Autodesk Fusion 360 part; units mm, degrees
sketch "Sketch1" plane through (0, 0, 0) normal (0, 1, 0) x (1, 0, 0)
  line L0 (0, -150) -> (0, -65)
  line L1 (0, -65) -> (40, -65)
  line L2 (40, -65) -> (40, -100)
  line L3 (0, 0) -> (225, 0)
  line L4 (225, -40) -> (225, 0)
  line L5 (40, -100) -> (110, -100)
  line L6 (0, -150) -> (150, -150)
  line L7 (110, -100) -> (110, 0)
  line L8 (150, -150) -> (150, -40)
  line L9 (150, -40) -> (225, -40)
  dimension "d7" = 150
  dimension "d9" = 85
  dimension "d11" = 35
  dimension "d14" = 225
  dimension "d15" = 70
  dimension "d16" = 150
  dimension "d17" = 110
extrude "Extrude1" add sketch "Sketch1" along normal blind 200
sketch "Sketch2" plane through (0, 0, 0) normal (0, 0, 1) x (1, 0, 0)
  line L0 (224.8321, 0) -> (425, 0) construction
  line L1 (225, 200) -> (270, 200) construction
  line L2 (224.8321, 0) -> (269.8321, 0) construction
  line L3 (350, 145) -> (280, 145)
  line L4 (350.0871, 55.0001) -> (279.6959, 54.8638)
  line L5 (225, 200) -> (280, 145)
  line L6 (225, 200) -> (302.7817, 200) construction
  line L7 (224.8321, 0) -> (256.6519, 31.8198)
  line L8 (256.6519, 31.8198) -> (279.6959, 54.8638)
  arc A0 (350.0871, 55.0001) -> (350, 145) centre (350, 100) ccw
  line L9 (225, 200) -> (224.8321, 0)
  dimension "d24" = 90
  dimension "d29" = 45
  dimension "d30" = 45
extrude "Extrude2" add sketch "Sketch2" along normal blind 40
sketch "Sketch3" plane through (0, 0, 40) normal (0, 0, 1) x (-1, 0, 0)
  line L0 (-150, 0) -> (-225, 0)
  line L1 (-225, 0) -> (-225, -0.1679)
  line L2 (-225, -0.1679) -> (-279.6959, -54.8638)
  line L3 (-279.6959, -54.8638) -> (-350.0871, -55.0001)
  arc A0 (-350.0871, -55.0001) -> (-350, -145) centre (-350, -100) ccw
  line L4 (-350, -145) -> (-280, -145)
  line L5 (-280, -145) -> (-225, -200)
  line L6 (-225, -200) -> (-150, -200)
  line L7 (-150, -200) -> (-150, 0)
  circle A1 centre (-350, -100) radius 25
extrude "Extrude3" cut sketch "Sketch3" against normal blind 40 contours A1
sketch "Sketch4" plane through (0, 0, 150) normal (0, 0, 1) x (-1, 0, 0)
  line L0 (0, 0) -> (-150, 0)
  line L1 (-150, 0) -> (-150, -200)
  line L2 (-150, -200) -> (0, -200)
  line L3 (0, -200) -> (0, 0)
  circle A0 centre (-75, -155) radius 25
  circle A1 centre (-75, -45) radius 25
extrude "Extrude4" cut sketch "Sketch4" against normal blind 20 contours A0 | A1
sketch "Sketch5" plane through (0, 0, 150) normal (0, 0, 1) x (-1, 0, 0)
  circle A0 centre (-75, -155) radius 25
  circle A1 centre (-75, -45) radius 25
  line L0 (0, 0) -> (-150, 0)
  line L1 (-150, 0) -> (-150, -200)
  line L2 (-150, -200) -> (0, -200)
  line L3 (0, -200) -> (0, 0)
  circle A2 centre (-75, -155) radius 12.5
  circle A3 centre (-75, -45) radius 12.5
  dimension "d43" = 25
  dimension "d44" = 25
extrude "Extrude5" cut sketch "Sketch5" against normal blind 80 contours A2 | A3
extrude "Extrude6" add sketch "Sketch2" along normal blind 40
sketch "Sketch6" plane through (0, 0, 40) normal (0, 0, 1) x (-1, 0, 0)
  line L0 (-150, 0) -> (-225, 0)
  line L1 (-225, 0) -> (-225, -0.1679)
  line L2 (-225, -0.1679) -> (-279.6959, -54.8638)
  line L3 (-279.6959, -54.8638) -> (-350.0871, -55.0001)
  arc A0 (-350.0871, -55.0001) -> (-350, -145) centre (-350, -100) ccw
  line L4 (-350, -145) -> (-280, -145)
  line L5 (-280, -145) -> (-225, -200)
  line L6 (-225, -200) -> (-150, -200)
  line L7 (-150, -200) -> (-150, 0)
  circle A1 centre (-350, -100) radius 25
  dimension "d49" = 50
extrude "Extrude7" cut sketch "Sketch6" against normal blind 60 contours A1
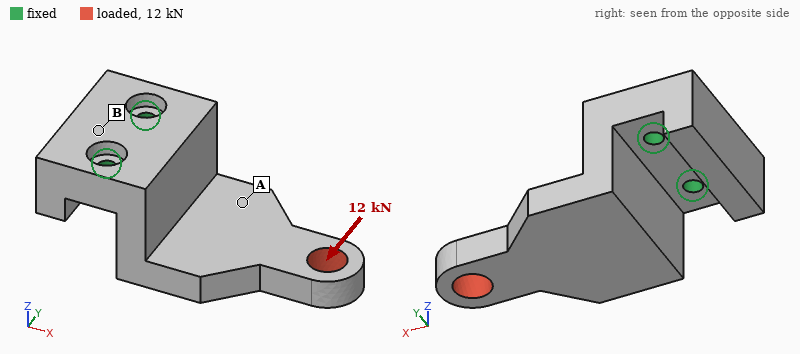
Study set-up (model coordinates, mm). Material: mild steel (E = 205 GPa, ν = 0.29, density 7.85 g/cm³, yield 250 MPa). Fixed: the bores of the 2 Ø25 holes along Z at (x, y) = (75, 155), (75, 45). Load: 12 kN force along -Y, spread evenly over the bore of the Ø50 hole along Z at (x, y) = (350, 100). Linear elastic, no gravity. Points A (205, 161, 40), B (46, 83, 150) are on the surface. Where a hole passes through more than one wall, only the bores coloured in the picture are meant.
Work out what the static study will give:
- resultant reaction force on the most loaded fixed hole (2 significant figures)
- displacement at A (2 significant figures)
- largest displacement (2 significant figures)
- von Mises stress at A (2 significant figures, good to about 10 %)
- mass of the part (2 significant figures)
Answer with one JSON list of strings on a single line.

["29 kN", "0.046 mm", "0.15 mm", "13 MPa", "29 kg"]
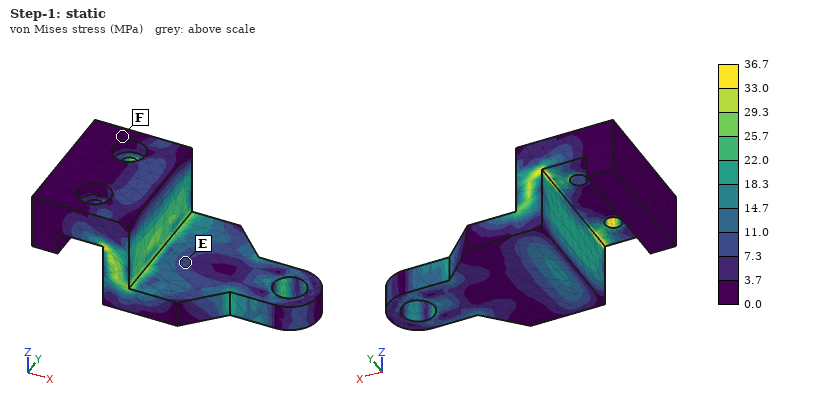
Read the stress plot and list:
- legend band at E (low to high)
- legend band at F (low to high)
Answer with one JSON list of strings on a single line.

["7.3 to 11.0 MPa", "0.0 to 3.7 MPa"]
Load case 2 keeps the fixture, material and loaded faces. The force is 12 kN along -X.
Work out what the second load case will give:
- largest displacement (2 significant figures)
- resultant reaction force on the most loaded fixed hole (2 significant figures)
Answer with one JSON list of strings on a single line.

["0.16 mm", "6.2 kN"]
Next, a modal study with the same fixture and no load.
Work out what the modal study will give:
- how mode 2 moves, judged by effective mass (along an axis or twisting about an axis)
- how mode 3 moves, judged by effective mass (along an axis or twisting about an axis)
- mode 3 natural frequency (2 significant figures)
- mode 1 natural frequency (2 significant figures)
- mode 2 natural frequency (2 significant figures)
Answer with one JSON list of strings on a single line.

["along Y", "along X", "1200 Hz", "360 Hz", "870 Hz"]
